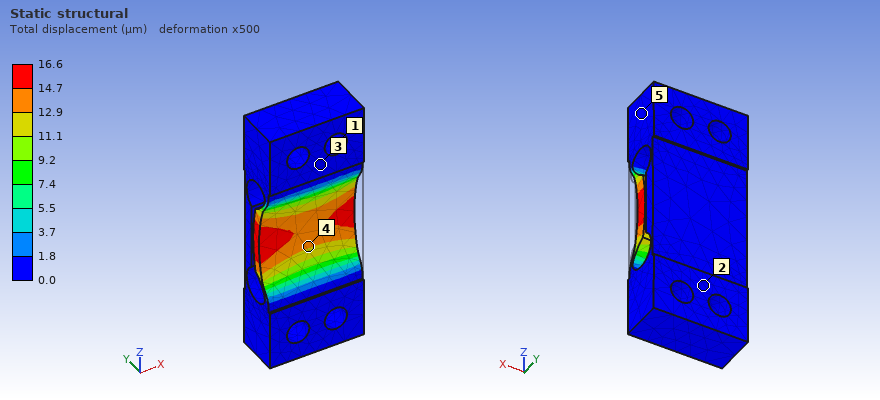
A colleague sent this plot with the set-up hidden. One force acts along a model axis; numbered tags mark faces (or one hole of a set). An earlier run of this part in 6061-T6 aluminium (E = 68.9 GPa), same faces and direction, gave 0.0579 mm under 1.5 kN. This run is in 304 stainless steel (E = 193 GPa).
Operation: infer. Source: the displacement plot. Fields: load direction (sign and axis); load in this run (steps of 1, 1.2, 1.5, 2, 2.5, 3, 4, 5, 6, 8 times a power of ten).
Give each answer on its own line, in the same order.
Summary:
+Y
1.2 kN
